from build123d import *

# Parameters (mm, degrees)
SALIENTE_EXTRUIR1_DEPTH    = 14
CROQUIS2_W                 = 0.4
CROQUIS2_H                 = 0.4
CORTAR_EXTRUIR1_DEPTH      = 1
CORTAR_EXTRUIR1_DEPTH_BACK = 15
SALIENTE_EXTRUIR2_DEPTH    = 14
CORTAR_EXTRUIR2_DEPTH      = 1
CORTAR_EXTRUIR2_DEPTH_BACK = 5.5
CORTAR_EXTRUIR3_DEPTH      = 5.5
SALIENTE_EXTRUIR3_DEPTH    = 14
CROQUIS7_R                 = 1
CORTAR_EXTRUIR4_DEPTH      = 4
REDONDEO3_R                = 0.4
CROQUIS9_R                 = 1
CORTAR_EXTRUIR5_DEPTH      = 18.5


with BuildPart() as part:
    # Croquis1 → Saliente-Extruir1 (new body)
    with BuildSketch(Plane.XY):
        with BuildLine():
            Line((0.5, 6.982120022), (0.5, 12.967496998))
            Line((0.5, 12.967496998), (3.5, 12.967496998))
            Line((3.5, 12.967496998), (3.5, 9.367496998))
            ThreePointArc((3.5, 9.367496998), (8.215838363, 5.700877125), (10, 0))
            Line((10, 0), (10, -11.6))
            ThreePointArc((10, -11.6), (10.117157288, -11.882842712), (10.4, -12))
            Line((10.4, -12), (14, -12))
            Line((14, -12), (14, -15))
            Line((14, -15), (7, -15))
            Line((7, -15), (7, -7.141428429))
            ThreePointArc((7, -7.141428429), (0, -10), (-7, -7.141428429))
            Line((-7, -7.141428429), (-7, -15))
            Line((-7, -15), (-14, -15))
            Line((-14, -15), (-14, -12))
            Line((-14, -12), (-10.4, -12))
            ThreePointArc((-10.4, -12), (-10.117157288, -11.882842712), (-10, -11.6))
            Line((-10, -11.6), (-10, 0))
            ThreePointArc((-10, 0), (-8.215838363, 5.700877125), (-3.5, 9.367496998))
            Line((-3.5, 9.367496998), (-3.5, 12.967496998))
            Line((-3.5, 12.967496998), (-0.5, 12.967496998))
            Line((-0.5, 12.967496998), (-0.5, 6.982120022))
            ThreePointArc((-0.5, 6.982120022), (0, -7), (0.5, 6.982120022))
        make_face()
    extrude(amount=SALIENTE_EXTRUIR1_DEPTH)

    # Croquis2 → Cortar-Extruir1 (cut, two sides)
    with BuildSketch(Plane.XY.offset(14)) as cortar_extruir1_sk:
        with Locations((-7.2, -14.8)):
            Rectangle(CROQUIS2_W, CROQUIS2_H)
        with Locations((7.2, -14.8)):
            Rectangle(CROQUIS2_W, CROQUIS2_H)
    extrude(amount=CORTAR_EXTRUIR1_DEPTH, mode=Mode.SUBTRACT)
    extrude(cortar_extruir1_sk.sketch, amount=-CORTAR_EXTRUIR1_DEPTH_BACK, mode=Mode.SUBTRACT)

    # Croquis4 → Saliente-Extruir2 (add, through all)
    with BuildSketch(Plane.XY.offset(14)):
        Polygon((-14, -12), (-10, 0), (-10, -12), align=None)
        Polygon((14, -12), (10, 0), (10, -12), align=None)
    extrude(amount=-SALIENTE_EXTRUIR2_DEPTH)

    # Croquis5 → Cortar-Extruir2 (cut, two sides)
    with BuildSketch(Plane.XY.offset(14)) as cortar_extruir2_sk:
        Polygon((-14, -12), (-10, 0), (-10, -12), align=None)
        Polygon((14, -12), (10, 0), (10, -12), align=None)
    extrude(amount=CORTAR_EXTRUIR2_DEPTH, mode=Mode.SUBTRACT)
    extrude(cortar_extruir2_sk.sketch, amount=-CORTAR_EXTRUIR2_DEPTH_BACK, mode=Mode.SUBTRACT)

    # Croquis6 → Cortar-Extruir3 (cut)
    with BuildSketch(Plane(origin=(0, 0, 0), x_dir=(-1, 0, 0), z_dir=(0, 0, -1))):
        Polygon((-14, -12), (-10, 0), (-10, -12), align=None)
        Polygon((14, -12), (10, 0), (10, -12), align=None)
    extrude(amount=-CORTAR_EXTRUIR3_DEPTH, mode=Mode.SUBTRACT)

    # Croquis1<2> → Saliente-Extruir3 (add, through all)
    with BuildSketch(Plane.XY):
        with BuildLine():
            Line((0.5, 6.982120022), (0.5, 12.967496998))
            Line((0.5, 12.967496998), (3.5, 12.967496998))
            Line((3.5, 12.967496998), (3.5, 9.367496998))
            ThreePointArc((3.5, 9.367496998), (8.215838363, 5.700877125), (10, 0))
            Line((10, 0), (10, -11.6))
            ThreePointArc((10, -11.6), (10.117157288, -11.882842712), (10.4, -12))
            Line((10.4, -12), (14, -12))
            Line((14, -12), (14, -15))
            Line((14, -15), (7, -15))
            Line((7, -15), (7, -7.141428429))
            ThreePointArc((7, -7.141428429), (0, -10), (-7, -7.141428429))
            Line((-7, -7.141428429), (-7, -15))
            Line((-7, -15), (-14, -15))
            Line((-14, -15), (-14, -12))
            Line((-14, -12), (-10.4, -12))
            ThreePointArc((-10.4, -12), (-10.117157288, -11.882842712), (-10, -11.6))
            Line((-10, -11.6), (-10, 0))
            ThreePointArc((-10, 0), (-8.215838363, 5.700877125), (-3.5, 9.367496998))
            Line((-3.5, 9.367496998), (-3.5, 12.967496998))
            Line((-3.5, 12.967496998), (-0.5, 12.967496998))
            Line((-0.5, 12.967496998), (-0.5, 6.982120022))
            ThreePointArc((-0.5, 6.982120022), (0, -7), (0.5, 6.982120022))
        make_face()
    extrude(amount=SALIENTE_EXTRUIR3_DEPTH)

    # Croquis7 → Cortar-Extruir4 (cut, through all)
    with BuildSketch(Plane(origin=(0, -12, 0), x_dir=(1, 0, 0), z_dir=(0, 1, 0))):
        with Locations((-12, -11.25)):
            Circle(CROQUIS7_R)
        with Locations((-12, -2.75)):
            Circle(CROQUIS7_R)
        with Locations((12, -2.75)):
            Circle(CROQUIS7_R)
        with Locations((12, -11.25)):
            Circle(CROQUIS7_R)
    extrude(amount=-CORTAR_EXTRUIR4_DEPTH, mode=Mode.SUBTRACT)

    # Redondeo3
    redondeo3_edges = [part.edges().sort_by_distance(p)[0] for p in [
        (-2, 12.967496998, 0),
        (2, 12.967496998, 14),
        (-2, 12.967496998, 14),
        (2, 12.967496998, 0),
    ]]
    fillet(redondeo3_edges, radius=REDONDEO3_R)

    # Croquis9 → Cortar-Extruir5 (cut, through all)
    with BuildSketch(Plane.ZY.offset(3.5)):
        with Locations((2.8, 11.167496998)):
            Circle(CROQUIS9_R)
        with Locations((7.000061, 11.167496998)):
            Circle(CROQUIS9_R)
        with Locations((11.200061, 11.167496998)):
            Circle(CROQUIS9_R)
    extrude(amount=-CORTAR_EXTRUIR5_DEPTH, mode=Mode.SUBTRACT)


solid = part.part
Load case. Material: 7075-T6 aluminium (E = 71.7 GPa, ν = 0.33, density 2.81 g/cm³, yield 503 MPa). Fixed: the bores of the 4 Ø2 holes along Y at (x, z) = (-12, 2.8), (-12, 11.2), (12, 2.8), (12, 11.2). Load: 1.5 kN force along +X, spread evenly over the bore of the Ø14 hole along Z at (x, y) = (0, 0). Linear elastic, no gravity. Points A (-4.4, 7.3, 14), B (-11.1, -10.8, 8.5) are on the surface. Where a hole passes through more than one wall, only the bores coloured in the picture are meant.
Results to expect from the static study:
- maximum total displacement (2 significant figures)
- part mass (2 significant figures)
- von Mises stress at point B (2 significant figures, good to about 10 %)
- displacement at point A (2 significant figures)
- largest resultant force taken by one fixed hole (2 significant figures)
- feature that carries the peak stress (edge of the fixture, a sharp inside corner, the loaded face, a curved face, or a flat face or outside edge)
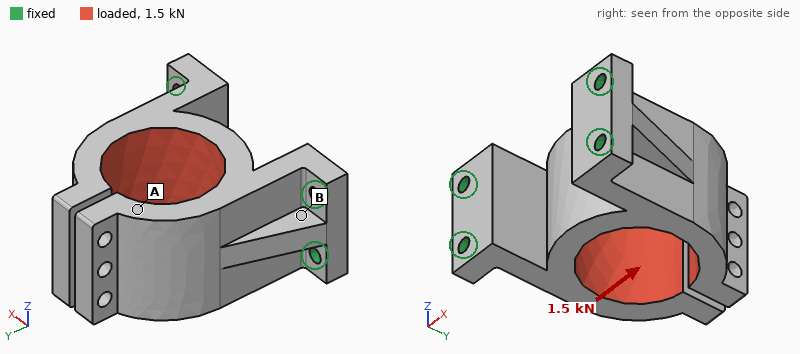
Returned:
0.18 mm
10 g
62 MPa
0.12 mm
500 N
a curved face
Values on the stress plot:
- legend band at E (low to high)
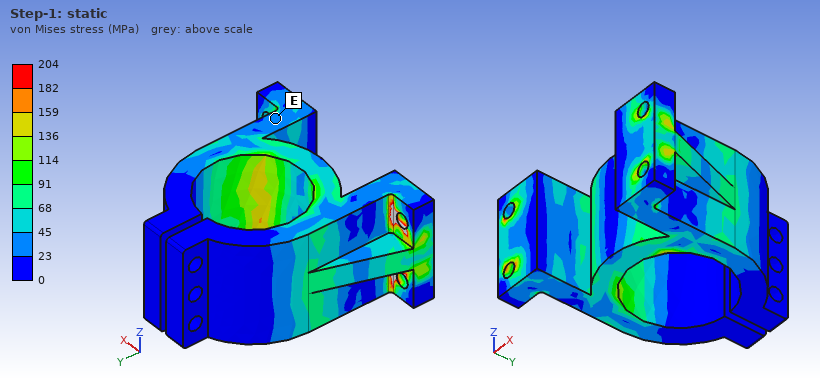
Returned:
23 to 45 MPa
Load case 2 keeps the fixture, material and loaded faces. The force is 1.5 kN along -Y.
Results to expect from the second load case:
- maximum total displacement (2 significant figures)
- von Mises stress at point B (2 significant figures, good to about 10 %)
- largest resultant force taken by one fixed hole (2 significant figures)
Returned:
0.13 mm
18 MPa
440 N
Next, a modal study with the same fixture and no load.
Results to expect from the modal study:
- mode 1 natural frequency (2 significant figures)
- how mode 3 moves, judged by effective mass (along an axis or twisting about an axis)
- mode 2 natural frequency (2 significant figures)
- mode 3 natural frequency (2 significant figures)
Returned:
5700 Hz
along Z
5900 Hz
8500 Hz
